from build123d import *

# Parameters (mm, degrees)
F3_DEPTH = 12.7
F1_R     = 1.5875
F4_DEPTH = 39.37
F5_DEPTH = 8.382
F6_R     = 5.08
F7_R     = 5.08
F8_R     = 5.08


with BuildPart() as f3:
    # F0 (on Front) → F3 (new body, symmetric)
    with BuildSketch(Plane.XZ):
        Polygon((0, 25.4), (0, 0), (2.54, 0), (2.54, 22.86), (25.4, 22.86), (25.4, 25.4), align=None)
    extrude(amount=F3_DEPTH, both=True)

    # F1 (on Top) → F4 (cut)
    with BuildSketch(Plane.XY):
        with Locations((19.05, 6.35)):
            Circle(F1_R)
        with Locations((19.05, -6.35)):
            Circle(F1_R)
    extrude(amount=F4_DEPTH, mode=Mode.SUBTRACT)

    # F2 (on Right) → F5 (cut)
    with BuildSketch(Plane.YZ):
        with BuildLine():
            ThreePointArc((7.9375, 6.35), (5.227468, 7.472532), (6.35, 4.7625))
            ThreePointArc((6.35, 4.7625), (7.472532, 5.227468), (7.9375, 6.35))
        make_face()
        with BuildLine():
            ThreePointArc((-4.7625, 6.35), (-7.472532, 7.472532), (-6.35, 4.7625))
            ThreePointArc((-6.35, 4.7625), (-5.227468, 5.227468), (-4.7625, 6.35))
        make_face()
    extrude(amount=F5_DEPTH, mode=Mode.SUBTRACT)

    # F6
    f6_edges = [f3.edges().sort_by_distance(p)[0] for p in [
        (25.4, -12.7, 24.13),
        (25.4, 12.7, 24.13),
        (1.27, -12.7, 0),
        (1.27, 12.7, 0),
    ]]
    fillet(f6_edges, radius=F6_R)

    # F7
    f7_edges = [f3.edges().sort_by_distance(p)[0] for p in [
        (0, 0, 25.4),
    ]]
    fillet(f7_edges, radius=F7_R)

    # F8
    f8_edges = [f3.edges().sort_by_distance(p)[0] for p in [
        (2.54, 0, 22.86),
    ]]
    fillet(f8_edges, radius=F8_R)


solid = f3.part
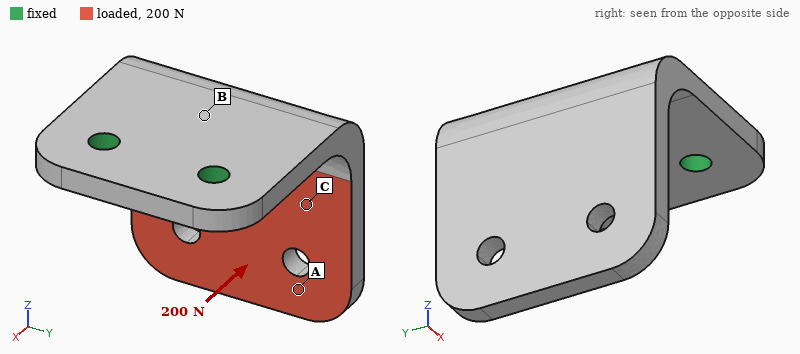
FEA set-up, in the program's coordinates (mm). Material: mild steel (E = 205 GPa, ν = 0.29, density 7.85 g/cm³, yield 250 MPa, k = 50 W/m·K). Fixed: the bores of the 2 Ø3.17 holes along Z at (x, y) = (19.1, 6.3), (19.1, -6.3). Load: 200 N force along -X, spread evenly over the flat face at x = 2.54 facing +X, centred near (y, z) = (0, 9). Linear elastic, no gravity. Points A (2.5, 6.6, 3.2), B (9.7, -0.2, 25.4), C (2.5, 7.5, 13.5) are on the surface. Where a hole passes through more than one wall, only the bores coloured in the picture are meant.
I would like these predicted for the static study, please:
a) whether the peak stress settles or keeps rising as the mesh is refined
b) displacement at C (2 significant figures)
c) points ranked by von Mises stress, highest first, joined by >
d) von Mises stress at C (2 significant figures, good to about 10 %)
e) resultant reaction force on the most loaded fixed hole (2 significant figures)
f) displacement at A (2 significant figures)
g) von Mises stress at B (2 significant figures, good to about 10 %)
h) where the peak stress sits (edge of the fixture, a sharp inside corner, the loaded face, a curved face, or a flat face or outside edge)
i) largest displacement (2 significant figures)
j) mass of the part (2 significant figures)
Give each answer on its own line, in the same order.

keeps rising
0.084 mm
B > C > A
34 MPa
100 N
0.16 mm
95 MPa
edge of the fixture
0.19 mm
23 g
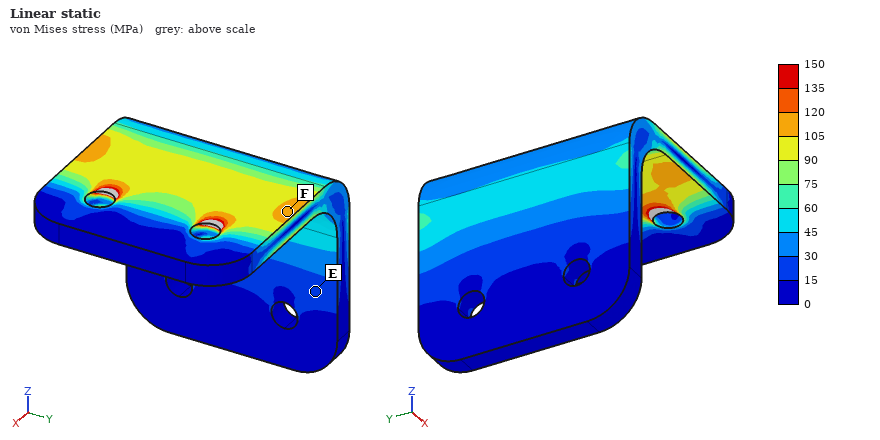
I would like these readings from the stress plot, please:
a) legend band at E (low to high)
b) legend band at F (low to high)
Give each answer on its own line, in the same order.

15 to 30 MPa
105 to 120 MPa
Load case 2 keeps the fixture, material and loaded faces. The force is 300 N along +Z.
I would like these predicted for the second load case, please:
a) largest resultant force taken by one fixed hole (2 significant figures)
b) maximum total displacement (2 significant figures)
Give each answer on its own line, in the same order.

150 N
0.14 mm
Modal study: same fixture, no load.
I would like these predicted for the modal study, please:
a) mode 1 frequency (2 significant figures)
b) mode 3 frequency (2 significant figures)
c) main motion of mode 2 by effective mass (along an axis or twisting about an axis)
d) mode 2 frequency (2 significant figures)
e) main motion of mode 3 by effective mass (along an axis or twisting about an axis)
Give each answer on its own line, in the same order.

1800 Hz
5900 Hz
along Y
3400 Hz
along Z
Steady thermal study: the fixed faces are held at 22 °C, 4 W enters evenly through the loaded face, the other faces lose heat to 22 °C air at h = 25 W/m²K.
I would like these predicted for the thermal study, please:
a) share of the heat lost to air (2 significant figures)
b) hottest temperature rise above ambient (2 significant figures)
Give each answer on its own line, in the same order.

19 %
31 K
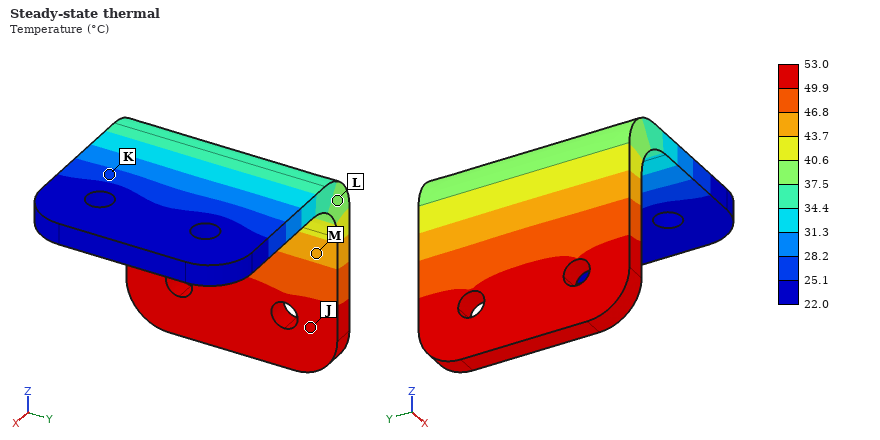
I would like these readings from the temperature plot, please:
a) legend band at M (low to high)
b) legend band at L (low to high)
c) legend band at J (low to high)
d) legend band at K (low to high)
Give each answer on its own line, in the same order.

43.7 to 46.8 °C
37.5 to 40.6 °C
49.9 to 53.0 °C
25.1 to 28.2 °C
